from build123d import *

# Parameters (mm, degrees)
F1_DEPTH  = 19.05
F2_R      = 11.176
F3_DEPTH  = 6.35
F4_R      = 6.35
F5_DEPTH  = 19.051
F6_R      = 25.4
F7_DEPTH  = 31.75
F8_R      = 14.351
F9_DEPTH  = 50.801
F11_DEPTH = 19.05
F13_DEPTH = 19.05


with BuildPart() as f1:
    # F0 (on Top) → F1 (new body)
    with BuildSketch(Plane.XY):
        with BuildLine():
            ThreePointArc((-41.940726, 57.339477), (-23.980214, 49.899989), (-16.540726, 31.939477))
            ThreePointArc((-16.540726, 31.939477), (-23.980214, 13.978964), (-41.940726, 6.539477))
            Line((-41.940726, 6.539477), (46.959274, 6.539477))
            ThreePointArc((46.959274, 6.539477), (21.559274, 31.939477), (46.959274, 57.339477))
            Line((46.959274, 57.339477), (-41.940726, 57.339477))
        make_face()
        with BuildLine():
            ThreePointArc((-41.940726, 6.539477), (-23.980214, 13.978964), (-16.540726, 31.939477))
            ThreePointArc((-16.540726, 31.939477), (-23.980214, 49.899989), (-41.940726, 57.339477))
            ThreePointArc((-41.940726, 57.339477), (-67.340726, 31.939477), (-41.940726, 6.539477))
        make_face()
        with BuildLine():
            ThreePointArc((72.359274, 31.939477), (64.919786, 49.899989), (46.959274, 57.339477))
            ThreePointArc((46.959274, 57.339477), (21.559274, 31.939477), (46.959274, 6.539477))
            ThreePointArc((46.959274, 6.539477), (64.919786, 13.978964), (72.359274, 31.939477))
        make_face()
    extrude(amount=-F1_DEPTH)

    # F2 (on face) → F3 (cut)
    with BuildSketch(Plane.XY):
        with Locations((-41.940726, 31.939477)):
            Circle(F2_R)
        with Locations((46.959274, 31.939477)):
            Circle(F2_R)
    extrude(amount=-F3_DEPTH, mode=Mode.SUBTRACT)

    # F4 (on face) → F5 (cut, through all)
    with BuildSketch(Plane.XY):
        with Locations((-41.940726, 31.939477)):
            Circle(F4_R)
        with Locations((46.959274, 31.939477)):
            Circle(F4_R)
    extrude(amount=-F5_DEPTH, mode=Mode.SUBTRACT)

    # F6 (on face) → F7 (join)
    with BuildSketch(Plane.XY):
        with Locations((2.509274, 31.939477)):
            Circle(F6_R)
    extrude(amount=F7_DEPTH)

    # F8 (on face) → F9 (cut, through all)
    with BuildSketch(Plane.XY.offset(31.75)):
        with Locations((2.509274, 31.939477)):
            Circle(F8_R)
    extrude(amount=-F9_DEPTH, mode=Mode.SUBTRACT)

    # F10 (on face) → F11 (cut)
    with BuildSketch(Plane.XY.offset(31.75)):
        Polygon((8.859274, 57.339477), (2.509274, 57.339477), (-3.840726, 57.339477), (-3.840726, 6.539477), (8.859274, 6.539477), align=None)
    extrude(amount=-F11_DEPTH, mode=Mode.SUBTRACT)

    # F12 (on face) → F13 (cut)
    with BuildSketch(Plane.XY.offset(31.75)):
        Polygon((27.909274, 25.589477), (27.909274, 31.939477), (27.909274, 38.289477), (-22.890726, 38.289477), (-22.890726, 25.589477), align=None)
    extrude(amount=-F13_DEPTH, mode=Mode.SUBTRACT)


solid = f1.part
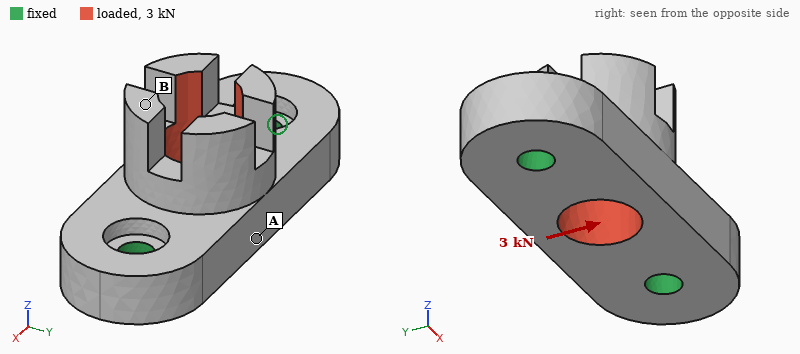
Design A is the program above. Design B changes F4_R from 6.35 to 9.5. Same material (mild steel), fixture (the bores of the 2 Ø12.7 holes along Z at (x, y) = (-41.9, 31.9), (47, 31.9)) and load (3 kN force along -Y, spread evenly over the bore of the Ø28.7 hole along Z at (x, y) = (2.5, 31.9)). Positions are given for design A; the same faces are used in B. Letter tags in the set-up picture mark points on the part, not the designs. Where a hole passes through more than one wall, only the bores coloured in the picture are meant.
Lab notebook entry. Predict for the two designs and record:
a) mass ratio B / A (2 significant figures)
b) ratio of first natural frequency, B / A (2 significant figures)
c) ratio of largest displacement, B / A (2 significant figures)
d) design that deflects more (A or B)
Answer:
0.97
1.2
0.73
A
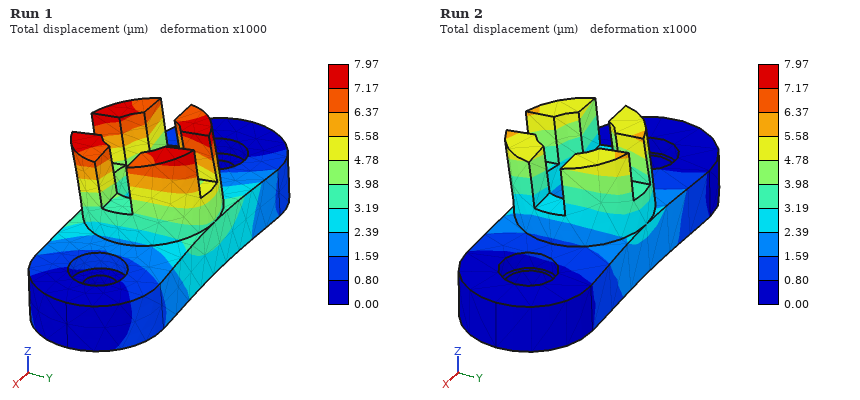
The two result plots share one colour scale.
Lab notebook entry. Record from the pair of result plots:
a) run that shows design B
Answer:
Run 2
